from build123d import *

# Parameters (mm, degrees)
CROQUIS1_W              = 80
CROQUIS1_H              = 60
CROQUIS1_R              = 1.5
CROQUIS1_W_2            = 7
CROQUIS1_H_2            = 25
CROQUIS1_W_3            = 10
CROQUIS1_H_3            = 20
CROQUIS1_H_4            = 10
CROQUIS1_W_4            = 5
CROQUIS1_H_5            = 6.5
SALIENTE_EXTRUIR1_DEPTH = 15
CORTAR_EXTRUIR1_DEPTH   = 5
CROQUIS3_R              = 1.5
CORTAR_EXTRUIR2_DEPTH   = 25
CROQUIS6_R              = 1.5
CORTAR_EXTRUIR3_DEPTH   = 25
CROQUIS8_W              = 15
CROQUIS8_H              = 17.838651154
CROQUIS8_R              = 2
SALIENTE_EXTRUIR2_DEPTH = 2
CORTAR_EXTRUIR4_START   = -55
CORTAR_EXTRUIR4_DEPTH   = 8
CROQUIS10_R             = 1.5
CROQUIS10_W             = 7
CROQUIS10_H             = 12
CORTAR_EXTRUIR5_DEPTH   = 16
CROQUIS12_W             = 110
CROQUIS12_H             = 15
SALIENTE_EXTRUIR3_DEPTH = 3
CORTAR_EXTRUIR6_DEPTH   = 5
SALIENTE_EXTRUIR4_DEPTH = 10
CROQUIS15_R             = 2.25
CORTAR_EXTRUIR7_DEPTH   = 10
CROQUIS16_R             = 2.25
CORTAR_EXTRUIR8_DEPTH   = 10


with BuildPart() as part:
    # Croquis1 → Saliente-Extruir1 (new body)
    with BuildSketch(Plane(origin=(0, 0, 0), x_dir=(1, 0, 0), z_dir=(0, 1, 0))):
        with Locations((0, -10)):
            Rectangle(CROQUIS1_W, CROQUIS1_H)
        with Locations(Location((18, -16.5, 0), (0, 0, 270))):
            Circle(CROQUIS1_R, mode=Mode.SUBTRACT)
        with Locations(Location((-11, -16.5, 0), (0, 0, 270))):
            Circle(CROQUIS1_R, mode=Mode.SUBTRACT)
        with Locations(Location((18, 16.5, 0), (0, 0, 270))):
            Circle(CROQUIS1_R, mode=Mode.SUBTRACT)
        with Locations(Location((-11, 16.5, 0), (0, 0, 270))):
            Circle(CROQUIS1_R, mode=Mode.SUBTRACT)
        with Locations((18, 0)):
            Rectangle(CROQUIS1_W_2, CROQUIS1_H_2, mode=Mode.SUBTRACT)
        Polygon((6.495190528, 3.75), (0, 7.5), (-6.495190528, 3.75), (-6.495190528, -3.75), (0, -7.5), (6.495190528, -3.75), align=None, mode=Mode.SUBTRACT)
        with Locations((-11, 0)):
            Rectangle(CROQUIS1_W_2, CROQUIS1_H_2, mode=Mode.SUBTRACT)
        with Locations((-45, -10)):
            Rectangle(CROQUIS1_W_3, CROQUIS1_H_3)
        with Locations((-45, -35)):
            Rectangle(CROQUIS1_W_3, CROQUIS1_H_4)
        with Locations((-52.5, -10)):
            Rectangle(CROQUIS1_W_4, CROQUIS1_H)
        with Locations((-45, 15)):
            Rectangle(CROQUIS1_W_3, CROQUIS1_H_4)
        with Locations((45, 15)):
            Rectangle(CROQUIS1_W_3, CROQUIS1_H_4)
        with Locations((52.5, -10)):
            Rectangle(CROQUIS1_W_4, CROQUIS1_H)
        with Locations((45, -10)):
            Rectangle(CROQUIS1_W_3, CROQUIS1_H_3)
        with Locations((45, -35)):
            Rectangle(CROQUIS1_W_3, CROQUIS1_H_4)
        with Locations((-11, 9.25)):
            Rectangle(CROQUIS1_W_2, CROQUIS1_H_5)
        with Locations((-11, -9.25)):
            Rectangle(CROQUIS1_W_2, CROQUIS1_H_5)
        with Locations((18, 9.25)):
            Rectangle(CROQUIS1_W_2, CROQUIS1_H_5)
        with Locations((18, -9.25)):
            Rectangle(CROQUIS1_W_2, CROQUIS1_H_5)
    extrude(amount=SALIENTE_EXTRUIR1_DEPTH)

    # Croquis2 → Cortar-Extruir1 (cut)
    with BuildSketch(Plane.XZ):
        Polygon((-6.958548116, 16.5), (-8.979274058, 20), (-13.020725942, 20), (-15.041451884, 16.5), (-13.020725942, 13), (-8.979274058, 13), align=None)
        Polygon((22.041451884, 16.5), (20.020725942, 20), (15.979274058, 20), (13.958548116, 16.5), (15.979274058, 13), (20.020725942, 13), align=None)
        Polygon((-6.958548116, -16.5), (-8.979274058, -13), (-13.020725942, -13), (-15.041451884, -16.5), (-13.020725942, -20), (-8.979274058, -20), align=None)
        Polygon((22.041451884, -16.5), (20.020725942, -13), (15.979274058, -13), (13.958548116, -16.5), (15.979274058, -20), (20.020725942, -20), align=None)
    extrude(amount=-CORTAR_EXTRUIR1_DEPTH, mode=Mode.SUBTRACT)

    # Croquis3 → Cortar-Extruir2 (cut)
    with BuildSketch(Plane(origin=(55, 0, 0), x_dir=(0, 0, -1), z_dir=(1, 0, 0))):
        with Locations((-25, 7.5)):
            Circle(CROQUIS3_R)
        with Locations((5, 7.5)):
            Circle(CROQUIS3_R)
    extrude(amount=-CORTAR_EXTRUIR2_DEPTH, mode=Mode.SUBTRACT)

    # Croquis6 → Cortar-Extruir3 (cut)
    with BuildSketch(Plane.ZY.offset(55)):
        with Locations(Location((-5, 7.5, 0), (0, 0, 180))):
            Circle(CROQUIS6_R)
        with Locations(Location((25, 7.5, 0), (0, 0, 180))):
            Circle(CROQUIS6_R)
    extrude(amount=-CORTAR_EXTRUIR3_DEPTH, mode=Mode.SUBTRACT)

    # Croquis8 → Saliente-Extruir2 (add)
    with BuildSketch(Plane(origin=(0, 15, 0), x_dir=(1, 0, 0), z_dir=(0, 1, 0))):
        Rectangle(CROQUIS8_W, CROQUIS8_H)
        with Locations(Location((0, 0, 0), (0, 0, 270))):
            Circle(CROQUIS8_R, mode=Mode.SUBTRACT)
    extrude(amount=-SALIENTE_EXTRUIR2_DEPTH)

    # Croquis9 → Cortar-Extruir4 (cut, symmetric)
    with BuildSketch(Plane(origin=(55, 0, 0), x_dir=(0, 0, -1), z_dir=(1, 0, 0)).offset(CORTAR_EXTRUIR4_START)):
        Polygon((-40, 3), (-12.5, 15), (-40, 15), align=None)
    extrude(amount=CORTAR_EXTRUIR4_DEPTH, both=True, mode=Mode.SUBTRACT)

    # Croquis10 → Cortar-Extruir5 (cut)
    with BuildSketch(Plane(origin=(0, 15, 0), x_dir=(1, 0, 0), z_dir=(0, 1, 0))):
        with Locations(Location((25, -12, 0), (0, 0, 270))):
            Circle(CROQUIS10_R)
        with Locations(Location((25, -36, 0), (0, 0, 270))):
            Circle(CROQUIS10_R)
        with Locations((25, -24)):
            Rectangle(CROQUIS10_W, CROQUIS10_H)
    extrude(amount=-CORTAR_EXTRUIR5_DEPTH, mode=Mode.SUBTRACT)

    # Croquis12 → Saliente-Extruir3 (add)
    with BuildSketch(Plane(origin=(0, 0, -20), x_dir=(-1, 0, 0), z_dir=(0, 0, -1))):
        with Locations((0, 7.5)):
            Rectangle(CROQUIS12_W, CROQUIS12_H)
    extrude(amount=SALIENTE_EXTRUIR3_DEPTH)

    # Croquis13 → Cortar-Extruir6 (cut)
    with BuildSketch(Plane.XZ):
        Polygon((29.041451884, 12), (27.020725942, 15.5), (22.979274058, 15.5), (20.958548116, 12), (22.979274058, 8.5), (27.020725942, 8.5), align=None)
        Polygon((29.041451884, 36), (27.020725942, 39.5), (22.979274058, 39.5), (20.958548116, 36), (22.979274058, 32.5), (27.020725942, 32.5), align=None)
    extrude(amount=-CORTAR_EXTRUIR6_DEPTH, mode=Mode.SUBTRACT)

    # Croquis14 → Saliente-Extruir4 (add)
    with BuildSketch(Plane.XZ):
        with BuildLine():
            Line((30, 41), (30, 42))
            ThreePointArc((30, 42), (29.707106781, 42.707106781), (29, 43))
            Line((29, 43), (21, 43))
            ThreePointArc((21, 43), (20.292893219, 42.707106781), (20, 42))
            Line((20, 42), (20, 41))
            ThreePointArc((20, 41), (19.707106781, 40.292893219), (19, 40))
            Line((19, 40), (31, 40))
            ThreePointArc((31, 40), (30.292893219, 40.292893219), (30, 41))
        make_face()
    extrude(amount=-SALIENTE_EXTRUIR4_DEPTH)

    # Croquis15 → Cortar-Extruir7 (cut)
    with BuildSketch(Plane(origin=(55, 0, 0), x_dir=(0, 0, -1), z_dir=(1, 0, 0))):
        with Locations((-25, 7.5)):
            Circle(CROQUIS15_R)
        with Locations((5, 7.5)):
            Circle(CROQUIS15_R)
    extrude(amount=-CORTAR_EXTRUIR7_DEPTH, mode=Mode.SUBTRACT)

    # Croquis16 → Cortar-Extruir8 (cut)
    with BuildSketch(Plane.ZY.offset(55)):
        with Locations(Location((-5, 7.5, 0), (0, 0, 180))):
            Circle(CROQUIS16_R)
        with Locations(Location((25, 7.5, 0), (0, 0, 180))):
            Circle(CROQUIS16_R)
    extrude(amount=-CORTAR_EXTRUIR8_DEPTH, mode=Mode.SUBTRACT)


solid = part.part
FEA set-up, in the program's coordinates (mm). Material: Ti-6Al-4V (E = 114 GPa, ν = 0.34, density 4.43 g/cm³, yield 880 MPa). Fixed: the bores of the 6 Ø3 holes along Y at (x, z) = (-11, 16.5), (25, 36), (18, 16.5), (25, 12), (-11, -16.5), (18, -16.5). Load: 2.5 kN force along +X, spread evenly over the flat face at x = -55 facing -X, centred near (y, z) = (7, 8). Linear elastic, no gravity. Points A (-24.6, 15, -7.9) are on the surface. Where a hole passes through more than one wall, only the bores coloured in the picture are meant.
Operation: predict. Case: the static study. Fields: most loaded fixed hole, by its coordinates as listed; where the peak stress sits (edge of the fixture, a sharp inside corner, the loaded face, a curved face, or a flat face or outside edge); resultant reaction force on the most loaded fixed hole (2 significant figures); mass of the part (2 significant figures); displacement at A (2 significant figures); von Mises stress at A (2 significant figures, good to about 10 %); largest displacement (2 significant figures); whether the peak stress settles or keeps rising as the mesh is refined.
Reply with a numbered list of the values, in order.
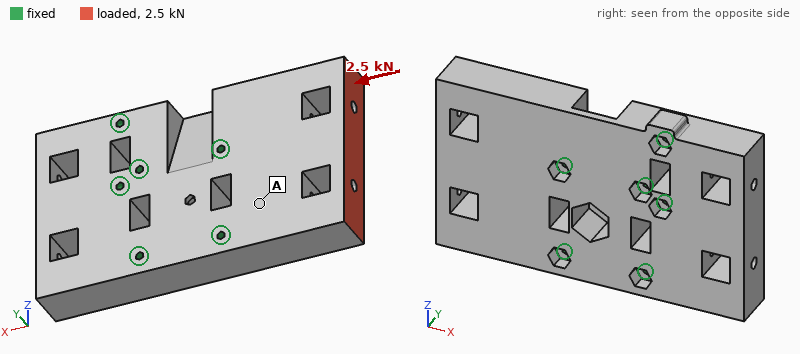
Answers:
1. (-11, 16.5)
2. edge of the fixture
3. 1.2 kN
4. 390 g
5. 0.60 µm
6. 2.1 MPa
7. 3.0 µm
8. keeps rising
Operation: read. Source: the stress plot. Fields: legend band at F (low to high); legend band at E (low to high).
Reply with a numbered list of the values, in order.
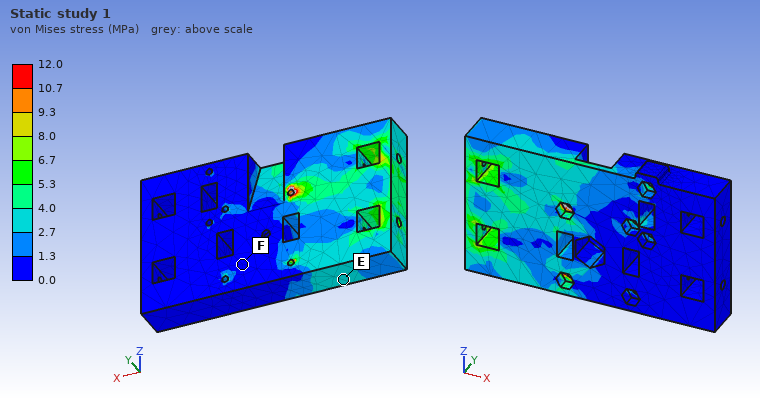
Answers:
1. 0.0 to 1.3 MPa
2. 2.7 to 4.0 MPa
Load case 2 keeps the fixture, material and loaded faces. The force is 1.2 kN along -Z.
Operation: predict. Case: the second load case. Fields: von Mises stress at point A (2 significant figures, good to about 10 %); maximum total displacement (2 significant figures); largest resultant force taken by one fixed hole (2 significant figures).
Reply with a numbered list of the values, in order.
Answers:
1. 5.3 MPa
2. 7.1 µm
3. 1.3 kN
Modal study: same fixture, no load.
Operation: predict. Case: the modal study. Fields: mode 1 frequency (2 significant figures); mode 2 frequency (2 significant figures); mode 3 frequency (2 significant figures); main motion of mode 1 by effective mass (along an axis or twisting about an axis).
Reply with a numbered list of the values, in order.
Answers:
1. 4100 Hz
2. 7000 Hz
3. 7200 Hz
4. along Y
